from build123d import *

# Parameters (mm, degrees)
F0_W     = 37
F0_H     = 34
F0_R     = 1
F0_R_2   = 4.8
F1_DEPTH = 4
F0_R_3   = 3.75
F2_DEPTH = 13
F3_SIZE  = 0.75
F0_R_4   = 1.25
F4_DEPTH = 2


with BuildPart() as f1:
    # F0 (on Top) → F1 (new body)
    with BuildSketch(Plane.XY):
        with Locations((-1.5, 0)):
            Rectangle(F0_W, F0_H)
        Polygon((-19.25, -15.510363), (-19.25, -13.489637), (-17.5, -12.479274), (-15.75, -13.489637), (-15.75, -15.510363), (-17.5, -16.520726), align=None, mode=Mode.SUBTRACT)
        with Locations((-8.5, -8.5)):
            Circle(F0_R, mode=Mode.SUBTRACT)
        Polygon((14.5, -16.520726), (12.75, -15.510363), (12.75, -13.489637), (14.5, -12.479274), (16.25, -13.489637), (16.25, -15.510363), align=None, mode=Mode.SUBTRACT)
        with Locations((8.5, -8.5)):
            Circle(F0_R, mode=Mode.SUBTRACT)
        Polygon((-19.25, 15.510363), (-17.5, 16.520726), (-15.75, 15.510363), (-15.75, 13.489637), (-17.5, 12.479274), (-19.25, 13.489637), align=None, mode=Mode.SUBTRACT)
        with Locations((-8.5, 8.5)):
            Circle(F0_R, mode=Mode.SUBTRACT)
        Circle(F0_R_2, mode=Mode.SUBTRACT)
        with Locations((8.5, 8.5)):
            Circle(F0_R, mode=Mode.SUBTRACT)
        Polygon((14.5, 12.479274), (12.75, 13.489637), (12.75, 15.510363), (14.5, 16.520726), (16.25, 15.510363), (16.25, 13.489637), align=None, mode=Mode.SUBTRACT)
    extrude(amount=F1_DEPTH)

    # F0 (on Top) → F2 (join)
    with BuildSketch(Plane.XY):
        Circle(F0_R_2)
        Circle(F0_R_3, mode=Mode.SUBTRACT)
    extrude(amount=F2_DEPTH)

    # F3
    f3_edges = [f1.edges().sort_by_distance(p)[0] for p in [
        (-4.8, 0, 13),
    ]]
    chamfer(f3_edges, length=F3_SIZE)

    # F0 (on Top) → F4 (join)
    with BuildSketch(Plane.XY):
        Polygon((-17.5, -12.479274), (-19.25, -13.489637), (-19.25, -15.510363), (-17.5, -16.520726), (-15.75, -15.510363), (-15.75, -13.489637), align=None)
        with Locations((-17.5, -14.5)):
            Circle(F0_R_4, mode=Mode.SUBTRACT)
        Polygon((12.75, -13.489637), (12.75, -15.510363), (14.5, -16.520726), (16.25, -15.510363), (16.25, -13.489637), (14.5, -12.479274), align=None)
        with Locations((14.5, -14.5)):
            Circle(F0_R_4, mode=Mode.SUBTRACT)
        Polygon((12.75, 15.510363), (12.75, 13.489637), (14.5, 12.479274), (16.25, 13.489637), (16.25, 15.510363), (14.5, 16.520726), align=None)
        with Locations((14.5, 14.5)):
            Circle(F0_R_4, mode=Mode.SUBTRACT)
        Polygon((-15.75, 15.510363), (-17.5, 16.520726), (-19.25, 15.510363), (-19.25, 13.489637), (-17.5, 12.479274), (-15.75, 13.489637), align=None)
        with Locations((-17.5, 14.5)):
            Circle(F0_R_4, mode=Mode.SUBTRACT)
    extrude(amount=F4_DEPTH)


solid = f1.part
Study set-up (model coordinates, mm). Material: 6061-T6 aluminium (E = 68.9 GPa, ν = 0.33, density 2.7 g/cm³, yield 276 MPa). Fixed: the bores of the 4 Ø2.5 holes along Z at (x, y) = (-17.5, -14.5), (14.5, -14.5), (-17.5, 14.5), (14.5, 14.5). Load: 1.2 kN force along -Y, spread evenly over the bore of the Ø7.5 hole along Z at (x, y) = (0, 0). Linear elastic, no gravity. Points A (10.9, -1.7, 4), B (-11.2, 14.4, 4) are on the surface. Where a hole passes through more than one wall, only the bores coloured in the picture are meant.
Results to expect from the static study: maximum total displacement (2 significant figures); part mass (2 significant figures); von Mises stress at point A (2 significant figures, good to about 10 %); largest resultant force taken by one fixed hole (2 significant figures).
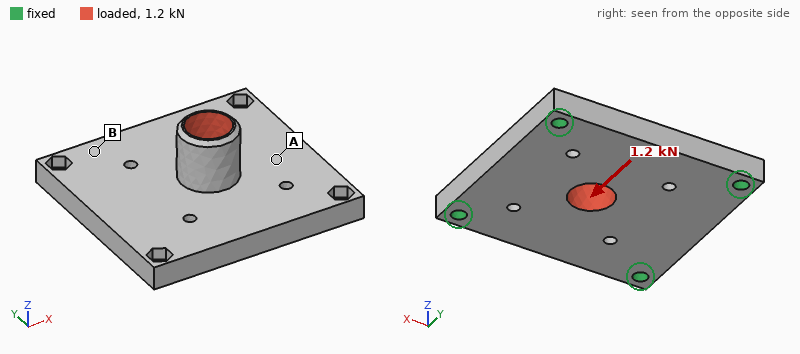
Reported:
42 µm
13 g
27 MPa
410 N
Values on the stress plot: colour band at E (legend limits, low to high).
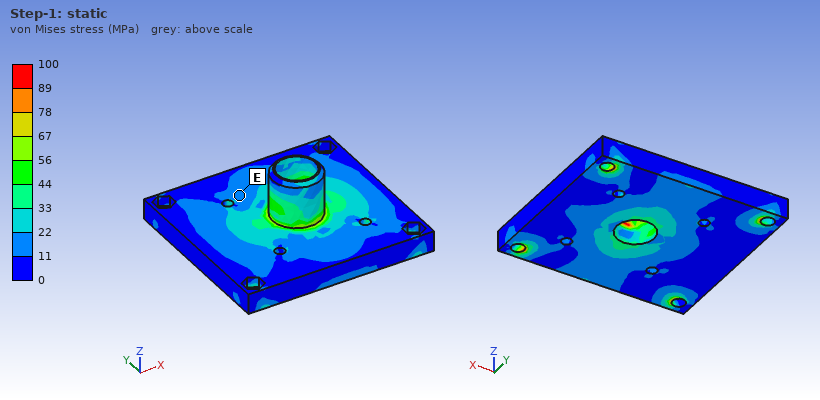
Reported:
11 to 22 MPa
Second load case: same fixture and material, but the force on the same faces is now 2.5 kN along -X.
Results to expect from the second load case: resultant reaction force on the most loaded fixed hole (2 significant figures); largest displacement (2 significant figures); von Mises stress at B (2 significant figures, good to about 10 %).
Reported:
780 N
84 µm
20 MPa
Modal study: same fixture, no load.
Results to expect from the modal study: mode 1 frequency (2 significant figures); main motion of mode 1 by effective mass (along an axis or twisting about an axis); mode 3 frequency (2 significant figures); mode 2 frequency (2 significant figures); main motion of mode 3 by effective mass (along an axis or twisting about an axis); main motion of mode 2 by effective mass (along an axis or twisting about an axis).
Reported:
11 kHz
along Z
19 kHz
17 kHz
twisting about Y
twisting about X
